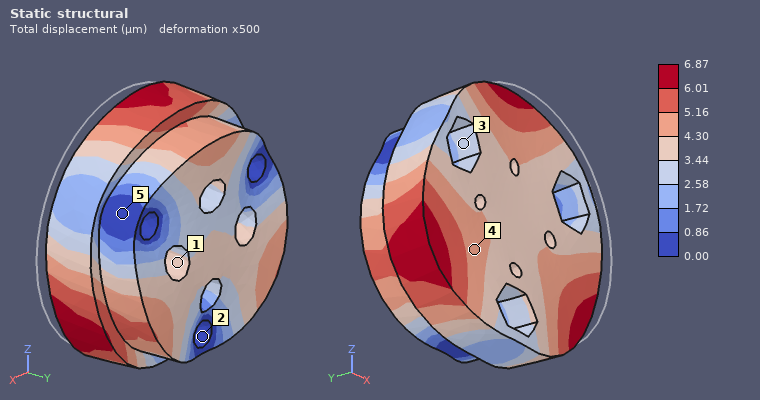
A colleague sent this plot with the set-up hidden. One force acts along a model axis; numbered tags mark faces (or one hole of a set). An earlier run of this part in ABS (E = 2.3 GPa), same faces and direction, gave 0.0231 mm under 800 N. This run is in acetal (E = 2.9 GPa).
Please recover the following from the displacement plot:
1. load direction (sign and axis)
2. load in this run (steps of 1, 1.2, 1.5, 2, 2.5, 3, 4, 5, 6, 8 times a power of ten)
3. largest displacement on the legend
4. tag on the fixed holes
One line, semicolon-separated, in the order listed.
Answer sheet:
+Y; 300 N; 6.87 µm; 2
